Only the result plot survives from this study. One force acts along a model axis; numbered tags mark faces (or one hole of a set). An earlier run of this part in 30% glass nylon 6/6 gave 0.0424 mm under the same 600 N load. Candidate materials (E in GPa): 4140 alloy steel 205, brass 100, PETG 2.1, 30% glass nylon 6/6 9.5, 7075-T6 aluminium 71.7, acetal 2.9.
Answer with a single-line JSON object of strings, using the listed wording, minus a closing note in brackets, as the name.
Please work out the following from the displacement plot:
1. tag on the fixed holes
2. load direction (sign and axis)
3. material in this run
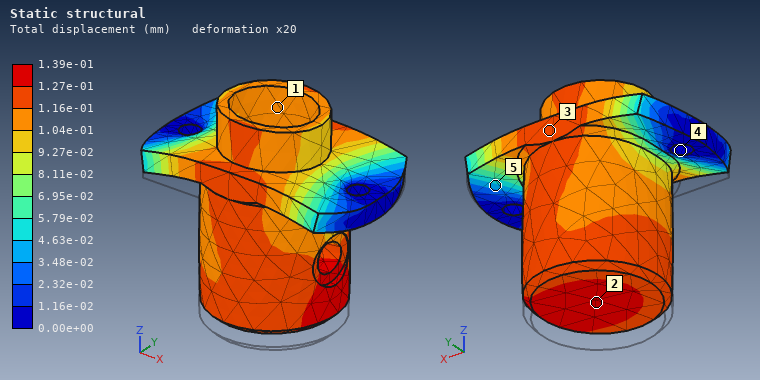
{"tag on the fixed holes": "4", "load direction": "+Z", "material in this run": "acetal"}
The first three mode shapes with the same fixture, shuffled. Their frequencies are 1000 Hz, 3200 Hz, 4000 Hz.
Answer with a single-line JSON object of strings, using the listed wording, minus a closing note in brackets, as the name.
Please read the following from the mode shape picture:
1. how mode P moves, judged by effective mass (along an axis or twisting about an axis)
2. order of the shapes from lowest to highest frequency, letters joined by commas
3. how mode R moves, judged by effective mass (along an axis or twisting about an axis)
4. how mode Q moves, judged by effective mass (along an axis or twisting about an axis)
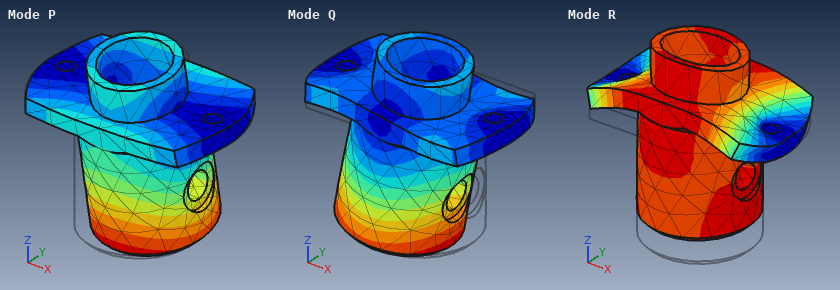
{"how mode P moves, judged by effective mass": "along Y", "order of the shapes from lowest to highest frequency, letters joined by commas": "P, Q, R", "how mode R moves, judged by effective mass": "along Z", "how mode Q moves, judged by effective mass": "along X"}
